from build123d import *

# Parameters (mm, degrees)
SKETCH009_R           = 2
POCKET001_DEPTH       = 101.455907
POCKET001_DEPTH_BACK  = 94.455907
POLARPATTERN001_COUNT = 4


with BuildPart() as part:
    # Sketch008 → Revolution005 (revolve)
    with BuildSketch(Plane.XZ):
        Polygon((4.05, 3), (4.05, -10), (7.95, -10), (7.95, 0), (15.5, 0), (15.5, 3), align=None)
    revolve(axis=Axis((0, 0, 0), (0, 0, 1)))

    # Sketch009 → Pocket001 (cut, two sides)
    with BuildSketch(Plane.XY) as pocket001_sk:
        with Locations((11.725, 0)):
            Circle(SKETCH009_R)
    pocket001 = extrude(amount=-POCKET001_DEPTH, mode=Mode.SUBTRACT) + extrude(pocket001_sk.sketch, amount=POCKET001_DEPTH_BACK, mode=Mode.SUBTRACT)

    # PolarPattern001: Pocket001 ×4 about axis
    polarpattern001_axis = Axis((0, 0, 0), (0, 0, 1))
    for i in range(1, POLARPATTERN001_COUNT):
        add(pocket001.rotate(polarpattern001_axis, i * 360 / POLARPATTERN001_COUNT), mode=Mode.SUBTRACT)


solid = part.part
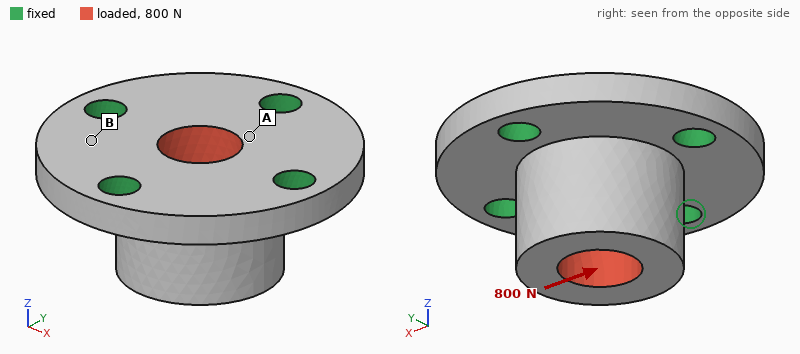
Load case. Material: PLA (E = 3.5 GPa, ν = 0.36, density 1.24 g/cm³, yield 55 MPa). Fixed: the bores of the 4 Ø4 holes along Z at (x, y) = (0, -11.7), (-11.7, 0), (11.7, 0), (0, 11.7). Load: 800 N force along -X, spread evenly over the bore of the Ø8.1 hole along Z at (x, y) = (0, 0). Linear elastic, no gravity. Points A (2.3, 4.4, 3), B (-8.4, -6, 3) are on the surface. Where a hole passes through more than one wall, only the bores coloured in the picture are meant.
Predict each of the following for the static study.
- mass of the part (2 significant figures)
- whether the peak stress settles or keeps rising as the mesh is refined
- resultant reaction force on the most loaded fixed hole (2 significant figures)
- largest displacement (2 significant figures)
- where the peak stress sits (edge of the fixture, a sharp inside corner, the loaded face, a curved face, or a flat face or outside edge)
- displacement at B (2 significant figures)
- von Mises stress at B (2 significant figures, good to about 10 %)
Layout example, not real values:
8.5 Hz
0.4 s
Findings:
4.3 g
keeps rising
330 N
95 µm
edge of the fixture
21 µm
5.0 MPa
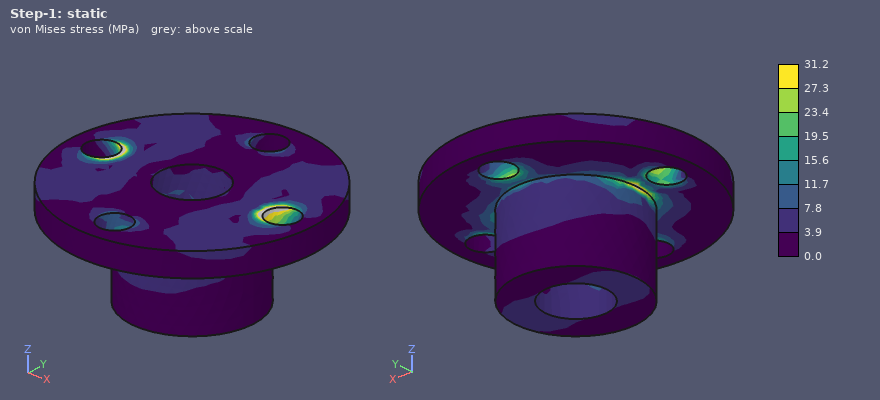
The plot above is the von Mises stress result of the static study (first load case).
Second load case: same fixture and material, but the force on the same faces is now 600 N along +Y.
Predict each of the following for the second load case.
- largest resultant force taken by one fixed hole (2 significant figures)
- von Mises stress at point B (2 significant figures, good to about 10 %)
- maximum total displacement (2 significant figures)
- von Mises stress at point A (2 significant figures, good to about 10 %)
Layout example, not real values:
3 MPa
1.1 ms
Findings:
250 N
3.4 MPa
71 µm
2.6 MPa
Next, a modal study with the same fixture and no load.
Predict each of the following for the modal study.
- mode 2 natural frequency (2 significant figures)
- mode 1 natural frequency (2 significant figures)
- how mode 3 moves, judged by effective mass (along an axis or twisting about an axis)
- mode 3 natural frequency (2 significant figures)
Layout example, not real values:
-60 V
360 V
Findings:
11 kHz
11 kHz
along Z
13 kHz
